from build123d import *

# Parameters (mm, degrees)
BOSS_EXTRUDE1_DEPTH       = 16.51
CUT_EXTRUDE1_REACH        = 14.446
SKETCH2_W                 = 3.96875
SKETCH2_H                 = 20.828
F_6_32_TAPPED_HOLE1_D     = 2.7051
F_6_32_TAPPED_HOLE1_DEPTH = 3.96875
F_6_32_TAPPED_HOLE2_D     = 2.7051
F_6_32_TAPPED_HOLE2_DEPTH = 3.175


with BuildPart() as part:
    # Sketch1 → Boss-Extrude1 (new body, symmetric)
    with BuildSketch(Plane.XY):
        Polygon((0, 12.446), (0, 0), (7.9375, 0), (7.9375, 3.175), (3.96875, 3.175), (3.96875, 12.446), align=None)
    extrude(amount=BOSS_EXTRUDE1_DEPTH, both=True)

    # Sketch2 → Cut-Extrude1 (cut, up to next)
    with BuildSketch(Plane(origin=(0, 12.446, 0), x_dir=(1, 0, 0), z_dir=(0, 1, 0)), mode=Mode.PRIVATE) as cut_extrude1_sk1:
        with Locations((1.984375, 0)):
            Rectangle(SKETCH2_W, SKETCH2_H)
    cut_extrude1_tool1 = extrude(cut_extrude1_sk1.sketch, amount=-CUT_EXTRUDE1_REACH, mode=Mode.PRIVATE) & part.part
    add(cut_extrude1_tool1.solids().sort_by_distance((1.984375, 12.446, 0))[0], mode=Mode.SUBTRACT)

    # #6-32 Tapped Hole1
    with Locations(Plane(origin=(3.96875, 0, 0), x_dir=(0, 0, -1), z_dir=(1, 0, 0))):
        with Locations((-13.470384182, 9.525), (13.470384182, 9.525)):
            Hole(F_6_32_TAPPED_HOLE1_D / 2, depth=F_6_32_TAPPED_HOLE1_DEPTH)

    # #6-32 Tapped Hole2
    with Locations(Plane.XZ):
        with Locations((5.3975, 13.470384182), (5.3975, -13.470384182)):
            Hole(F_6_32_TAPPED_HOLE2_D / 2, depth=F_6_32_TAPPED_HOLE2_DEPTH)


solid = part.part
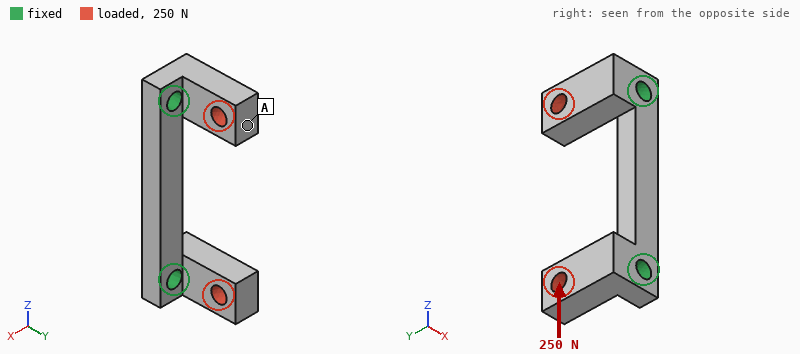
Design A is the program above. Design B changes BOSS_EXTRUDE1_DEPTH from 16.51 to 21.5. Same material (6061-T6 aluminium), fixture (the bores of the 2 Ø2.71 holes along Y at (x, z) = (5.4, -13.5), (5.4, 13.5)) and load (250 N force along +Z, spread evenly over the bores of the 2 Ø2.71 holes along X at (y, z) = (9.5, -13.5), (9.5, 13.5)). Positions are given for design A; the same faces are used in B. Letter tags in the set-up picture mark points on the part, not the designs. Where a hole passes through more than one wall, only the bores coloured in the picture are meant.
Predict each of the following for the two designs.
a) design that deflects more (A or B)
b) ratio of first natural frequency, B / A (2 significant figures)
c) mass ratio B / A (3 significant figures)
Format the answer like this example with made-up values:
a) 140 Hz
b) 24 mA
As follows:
a) A
b) 0.77
c) 1.66
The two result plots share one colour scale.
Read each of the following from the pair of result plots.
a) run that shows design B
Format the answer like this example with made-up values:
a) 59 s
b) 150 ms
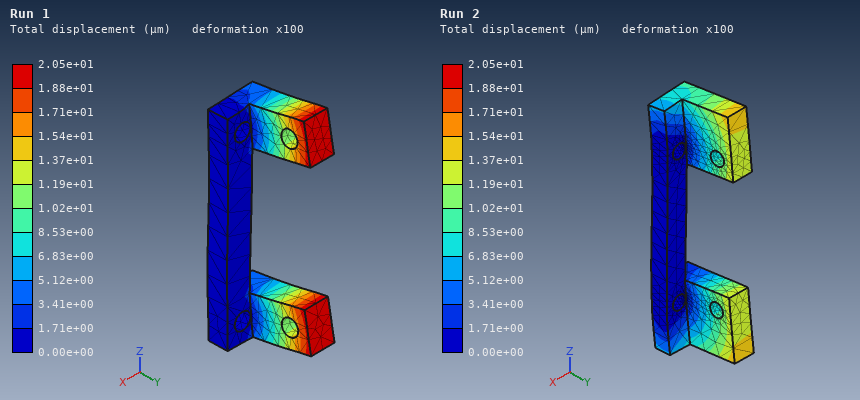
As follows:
a) Run 2
